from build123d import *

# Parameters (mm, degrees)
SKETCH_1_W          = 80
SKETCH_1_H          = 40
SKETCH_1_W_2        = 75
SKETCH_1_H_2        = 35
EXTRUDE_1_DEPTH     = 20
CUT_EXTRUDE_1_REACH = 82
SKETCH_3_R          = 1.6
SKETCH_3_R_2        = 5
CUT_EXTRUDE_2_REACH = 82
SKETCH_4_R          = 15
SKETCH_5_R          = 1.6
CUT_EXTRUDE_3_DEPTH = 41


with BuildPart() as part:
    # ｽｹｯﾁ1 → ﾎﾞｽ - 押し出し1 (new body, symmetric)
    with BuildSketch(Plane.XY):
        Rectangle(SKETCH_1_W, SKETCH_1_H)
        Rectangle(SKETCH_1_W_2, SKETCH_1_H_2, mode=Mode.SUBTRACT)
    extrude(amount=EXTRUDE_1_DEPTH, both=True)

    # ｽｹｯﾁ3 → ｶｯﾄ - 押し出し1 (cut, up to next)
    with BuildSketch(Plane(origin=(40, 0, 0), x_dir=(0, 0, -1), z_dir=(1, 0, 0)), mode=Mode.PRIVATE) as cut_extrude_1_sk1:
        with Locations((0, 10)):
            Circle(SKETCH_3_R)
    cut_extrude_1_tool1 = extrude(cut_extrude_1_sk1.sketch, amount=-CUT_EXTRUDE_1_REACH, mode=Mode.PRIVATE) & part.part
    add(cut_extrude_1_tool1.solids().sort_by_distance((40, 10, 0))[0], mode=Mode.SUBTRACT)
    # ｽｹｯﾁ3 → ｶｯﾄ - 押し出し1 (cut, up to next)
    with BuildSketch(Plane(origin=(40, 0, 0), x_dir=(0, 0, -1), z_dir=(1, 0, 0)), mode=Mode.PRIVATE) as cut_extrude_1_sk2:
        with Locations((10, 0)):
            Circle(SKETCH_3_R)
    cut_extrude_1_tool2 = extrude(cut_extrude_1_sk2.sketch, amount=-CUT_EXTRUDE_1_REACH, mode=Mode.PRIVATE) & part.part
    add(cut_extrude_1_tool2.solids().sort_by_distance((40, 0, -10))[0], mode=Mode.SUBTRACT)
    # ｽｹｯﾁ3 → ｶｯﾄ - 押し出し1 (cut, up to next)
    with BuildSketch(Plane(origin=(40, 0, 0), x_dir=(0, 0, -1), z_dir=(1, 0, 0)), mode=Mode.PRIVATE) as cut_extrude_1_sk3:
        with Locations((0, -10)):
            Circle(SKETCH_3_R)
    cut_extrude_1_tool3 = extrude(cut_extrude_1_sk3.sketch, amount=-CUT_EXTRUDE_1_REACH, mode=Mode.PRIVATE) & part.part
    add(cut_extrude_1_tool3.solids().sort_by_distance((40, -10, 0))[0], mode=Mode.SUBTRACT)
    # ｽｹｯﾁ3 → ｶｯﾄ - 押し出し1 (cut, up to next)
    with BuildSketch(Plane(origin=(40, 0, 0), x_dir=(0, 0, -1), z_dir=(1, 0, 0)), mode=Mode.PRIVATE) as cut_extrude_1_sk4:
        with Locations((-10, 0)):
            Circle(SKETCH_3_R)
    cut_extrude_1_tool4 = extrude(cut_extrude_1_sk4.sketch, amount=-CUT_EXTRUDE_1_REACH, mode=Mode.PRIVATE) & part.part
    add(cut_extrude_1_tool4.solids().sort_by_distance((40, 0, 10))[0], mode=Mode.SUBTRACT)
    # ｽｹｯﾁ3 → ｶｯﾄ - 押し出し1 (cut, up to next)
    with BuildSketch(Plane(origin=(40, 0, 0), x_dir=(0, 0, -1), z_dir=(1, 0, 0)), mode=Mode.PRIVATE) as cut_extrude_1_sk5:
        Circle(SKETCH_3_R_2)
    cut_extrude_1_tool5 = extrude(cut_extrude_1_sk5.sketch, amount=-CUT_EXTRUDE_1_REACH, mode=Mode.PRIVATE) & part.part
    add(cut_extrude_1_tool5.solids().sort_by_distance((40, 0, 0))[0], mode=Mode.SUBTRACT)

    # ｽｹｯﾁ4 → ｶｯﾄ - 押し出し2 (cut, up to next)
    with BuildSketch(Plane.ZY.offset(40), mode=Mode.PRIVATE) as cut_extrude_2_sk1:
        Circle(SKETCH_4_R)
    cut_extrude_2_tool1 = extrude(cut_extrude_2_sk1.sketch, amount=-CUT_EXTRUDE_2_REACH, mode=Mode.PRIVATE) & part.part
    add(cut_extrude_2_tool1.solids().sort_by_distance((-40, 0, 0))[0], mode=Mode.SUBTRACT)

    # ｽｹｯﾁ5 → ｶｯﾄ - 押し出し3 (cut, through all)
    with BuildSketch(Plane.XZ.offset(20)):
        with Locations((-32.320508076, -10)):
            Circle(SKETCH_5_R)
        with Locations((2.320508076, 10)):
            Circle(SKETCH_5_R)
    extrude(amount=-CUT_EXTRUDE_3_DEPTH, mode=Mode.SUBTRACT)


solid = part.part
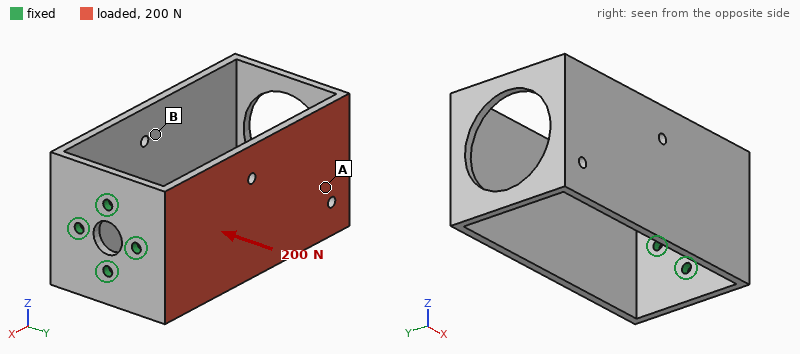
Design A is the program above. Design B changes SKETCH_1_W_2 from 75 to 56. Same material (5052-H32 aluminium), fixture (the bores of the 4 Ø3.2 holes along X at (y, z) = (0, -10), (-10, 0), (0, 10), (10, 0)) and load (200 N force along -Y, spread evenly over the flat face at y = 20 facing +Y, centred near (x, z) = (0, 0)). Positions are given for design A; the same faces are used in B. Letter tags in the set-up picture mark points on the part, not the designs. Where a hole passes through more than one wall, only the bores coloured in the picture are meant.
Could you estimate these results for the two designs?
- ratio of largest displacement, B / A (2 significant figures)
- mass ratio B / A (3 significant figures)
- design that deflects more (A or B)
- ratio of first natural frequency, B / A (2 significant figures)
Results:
0.22
1.90
A
1.5
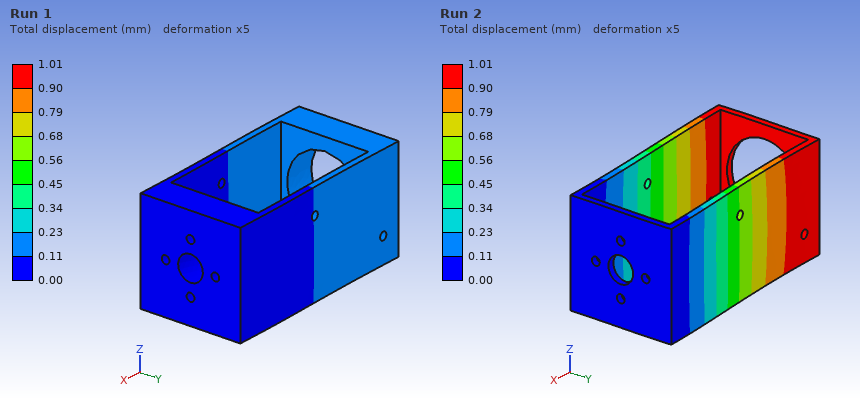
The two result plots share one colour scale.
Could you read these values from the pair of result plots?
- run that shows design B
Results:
Run 1
